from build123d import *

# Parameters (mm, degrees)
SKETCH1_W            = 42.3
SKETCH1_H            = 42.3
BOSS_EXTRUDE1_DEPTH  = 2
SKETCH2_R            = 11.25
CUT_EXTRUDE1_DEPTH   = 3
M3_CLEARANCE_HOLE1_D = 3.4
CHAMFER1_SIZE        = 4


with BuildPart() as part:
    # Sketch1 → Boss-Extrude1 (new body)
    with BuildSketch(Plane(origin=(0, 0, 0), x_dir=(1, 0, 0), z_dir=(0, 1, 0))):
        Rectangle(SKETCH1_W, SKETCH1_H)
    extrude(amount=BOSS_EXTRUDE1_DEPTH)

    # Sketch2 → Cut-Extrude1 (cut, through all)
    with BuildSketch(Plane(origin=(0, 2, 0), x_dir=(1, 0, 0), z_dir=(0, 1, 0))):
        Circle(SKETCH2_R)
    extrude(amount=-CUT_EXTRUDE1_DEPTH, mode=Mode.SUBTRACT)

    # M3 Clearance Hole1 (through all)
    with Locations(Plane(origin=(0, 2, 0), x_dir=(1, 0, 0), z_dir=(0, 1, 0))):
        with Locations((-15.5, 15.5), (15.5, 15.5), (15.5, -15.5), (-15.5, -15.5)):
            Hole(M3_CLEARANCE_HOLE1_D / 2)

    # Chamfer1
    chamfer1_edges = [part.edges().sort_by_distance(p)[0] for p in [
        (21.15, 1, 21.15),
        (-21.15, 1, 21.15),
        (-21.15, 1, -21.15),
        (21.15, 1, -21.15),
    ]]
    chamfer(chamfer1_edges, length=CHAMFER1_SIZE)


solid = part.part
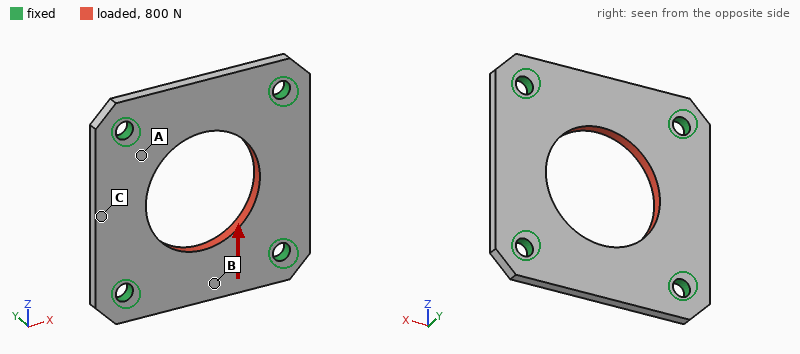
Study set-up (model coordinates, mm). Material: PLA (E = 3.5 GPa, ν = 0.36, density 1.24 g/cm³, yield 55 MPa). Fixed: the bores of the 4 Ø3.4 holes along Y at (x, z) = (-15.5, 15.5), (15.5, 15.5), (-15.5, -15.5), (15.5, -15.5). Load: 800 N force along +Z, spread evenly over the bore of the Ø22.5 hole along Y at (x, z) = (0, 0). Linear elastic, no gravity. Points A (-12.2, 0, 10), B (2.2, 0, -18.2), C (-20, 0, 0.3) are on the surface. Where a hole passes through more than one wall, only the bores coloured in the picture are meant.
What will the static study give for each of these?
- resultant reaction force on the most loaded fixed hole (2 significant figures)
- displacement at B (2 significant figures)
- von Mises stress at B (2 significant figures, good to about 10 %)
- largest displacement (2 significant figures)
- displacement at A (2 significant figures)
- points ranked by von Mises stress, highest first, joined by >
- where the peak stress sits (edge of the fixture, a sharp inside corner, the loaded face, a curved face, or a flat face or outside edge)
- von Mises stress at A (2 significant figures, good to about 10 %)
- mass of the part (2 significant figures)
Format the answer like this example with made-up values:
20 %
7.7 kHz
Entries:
210 N
65 µm
5.6 MPa
74 µm
23 µm
A > B > C
edge of the fixture
8.9 MPa
3.3 g
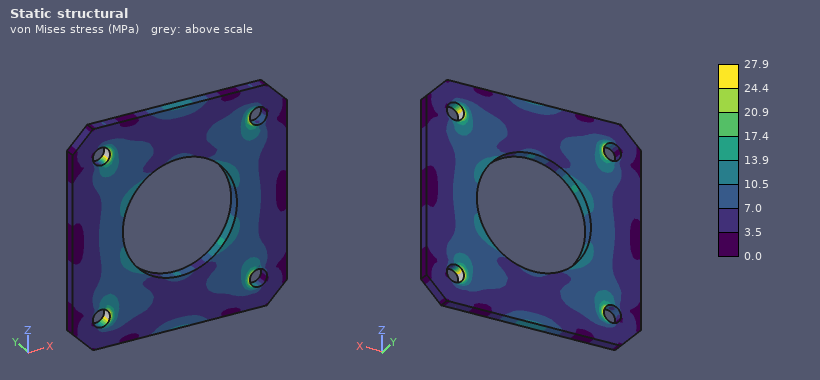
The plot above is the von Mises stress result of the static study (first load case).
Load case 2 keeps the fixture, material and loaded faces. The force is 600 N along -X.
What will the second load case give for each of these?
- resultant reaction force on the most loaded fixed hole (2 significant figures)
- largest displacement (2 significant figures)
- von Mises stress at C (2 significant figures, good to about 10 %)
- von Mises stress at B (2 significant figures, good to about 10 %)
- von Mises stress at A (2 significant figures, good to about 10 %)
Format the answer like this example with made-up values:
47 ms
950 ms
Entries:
150 N
55 µm
6.5 MPa
3.3 MPa
6.2 MPa
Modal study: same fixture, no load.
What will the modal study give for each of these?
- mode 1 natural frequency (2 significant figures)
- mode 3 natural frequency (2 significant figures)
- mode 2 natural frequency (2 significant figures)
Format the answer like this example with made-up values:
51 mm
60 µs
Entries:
4000 Hz
4100 Hz
4000 Hz
